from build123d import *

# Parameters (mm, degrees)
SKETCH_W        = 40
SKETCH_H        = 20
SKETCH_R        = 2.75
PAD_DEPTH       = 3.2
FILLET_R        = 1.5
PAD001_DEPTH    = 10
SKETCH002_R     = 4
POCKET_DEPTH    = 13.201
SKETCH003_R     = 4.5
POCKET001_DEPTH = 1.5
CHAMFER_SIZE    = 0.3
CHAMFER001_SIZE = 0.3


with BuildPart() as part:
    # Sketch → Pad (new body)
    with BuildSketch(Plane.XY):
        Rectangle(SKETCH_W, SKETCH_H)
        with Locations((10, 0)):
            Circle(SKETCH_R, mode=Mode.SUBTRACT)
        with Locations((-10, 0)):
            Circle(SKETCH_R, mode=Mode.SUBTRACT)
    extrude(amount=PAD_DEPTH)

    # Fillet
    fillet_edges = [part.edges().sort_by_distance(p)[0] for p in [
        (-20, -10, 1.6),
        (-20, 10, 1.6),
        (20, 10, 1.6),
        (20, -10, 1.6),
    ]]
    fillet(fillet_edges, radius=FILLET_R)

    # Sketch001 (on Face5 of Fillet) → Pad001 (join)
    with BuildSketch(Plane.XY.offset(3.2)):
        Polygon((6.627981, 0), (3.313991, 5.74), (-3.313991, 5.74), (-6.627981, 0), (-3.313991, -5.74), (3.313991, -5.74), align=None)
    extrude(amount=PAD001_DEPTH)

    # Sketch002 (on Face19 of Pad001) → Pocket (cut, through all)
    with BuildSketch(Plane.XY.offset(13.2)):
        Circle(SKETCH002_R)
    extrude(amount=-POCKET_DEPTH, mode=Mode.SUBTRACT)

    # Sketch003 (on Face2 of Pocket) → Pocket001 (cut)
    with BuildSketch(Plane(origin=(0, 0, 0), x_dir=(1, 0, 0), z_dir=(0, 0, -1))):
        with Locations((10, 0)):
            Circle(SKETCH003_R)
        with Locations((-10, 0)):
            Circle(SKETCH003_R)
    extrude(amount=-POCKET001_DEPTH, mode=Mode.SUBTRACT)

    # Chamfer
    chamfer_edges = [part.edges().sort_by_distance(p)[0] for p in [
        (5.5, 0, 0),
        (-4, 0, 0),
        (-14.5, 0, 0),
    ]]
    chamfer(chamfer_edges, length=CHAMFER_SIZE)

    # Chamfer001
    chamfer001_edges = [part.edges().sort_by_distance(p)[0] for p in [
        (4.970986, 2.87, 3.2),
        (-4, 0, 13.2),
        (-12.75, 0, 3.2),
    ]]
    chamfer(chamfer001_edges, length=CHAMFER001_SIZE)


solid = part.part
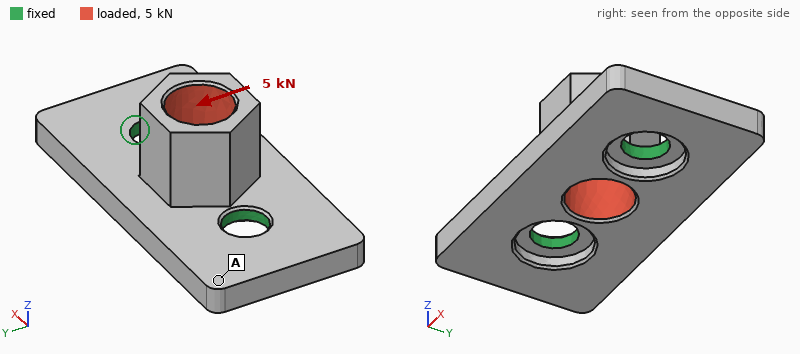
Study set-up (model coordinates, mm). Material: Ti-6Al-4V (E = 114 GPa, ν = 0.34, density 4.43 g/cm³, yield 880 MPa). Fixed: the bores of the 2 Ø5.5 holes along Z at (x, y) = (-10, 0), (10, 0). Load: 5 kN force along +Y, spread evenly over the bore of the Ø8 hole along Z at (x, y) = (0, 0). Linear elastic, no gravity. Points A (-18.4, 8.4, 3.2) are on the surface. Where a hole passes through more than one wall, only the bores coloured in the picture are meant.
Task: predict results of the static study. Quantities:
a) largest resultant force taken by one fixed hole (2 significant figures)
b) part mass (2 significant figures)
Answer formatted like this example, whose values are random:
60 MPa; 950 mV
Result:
2.5 kN; 12 g
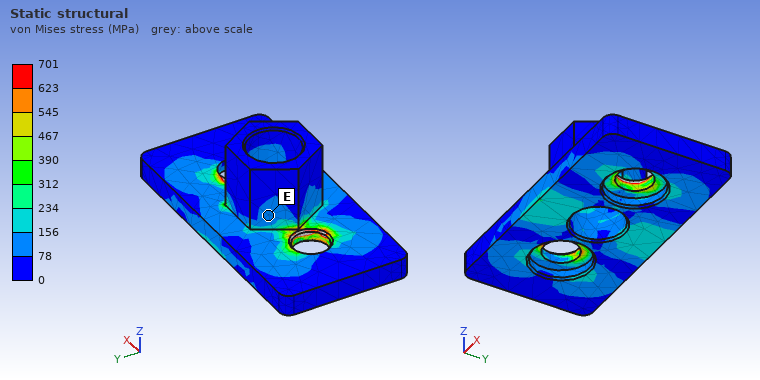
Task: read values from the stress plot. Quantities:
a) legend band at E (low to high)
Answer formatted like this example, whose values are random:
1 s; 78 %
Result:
78 to 156 MPa
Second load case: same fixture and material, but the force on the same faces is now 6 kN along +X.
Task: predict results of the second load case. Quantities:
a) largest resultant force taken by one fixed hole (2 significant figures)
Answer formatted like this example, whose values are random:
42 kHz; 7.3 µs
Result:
3.5 kN
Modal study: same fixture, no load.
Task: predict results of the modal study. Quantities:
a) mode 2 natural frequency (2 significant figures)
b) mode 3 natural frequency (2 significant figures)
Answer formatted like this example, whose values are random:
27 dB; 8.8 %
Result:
18 kHz; 18 kHz
